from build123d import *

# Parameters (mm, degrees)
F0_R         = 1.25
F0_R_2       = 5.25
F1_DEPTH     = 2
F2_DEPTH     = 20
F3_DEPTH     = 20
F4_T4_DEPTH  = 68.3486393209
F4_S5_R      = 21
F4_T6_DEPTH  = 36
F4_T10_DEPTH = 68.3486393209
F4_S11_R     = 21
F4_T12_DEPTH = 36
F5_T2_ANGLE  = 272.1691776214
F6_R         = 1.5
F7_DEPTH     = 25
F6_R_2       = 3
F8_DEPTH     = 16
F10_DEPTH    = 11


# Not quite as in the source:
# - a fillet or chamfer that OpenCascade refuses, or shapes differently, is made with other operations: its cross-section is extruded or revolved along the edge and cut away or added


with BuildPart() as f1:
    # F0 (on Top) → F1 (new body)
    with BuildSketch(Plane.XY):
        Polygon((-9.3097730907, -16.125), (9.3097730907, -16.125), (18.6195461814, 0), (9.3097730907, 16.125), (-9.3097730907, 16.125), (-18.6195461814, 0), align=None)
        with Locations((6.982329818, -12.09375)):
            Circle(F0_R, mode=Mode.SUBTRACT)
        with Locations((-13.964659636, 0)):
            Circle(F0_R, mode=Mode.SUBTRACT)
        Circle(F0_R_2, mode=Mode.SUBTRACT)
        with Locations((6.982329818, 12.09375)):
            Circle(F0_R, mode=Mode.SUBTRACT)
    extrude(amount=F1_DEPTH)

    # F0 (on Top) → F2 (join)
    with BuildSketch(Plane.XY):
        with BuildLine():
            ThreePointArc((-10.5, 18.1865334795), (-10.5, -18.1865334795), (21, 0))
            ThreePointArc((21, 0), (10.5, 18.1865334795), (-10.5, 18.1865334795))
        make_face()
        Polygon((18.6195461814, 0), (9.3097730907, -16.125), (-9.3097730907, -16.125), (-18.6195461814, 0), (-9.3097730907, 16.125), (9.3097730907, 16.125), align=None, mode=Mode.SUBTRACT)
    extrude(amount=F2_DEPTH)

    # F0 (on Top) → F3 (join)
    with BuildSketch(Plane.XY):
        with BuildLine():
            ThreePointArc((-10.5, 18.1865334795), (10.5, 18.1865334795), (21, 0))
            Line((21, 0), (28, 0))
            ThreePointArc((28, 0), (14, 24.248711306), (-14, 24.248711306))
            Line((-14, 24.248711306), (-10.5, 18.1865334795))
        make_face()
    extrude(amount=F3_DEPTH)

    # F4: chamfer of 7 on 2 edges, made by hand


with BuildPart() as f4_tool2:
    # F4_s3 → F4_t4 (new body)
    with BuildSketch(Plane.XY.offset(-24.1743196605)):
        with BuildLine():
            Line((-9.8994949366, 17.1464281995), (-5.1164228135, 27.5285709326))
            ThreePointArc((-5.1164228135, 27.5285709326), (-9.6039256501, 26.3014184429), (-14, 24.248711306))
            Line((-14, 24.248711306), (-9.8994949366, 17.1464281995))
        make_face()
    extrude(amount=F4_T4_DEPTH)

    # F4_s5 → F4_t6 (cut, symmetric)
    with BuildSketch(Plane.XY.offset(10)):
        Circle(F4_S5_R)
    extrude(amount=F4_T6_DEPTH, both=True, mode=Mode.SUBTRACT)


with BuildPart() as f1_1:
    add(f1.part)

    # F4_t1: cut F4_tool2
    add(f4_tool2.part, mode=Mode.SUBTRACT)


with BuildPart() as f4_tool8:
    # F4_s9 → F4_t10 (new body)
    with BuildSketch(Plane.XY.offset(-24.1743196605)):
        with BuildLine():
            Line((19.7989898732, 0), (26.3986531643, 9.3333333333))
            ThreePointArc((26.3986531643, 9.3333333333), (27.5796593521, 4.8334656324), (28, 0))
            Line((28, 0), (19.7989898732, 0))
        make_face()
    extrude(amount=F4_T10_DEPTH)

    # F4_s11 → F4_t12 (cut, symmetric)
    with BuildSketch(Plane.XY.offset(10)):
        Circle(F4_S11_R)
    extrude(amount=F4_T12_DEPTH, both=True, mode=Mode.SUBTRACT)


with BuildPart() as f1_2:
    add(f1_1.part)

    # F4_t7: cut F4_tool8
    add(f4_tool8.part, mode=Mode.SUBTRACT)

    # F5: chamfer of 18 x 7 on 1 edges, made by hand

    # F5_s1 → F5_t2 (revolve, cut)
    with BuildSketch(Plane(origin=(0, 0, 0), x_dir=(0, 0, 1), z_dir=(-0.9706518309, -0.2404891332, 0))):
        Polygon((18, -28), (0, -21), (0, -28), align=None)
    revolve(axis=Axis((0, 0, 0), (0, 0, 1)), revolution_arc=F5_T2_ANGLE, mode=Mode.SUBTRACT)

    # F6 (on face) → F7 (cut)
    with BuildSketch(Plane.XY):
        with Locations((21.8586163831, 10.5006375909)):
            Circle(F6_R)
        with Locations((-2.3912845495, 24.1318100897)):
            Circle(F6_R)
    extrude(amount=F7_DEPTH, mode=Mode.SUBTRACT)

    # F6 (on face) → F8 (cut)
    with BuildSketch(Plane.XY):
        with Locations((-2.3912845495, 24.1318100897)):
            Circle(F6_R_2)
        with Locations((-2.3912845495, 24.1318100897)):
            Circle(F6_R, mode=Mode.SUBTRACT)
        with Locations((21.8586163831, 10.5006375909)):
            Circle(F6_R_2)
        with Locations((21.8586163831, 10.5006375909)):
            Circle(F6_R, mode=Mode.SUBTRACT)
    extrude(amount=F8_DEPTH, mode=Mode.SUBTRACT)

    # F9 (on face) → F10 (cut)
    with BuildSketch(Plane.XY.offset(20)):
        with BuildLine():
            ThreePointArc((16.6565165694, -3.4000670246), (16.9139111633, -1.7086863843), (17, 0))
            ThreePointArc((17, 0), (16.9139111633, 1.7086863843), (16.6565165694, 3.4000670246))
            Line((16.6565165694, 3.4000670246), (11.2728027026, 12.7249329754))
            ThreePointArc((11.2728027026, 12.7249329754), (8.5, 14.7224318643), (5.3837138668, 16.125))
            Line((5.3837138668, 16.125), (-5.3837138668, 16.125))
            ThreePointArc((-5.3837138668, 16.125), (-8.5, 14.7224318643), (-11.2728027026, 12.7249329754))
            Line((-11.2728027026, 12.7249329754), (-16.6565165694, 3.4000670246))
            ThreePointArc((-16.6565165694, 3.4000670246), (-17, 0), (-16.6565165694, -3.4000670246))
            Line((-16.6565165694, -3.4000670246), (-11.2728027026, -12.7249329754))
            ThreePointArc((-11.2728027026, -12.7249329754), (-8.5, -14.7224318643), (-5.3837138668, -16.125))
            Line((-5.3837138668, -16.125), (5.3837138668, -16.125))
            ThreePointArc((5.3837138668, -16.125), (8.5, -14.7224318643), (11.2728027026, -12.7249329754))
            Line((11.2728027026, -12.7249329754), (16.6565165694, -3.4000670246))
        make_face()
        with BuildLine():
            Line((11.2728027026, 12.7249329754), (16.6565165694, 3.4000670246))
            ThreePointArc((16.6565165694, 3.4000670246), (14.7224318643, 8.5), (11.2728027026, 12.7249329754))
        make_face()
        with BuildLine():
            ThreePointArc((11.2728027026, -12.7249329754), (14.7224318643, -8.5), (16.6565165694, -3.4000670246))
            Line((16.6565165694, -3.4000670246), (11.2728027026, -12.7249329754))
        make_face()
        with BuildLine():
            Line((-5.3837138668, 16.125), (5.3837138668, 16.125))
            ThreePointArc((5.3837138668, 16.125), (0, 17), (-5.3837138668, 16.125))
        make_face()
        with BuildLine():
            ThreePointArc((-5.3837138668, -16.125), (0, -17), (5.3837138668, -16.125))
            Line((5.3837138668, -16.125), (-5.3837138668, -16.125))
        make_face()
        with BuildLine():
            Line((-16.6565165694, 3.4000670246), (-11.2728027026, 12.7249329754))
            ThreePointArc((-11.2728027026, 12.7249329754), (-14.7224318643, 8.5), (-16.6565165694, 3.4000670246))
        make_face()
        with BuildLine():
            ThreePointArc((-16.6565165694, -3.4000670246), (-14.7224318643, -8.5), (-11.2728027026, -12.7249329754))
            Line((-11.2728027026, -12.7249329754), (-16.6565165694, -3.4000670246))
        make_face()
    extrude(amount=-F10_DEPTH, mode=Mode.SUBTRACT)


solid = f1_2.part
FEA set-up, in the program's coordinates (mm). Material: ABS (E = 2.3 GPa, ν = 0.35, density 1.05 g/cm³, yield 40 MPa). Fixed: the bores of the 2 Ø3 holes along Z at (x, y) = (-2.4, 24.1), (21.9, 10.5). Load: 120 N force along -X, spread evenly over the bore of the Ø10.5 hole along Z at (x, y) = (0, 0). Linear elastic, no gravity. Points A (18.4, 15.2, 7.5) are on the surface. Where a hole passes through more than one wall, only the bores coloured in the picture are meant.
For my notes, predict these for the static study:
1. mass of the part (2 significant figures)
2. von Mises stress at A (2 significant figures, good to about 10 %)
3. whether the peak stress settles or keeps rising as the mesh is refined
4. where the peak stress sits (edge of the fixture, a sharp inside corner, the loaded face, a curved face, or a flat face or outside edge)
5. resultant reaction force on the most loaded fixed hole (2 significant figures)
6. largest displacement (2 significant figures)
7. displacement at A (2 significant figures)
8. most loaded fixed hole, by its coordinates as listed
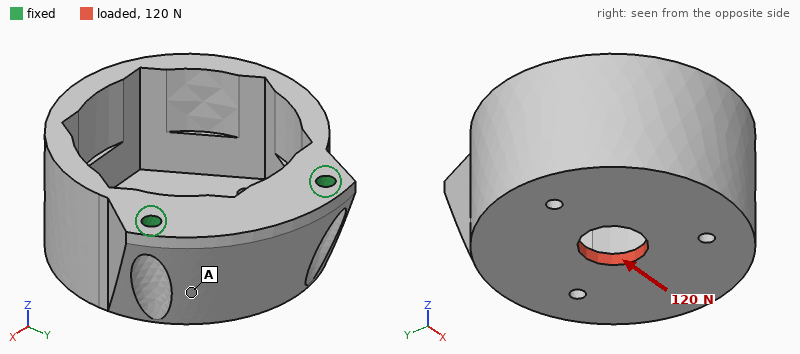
14 g
2.8 MPa
keeps rising
edge of the fixture
120 N
0.43 mm
0.10 mm
(21.9, 10.5)
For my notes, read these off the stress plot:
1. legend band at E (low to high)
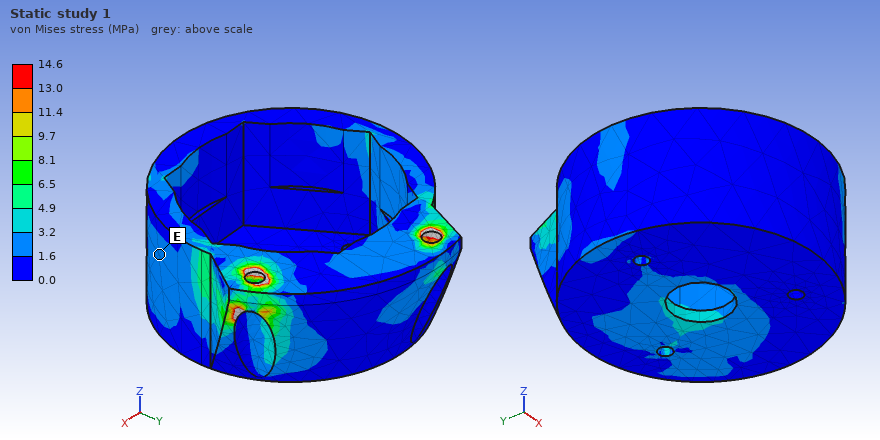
1.6 to 3.2 MPa
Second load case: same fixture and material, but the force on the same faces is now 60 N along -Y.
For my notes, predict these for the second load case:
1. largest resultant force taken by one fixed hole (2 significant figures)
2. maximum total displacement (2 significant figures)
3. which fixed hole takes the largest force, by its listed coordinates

50 N
0.33 mm
(-2.4, 24.1)
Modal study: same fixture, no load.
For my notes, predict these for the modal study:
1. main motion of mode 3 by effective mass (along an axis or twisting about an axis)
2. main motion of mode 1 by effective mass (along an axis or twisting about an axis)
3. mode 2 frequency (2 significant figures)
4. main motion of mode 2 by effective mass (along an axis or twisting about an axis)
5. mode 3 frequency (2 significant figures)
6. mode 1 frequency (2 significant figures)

along Y
along Z
960 Hz
along X
2400 Hz
620 Hz
